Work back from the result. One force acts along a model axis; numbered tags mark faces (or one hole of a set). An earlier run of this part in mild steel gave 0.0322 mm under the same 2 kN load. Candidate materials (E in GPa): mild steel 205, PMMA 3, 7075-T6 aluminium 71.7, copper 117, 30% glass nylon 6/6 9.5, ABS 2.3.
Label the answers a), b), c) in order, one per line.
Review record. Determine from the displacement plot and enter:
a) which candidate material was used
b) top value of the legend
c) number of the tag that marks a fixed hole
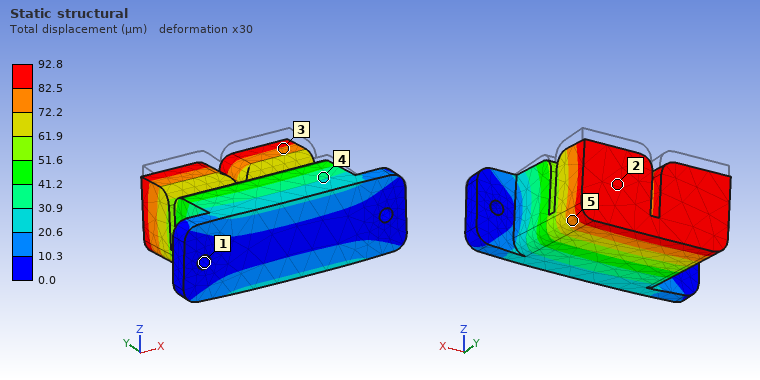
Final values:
a) 7075-T6 aluminium
b) 92.8 µm
c) 1
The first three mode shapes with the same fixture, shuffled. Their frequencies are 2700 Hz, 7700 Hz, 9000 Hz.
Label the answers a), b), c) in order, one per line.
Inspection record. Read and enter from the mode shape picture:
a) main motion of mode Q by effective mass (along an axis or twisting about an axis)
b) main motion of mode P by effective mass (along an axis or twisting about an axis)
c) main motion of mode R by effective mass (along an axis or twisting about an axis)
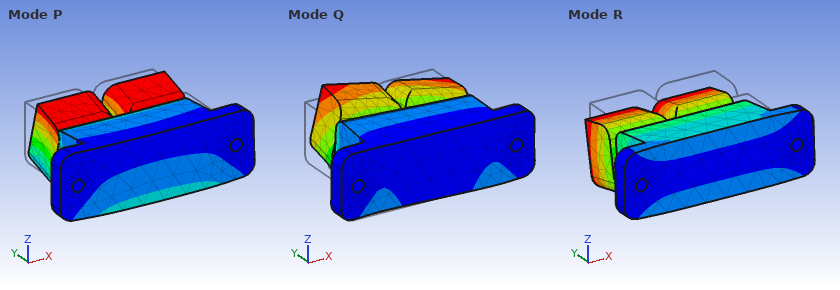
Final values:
a) along X
b) along Y
c) along Z
